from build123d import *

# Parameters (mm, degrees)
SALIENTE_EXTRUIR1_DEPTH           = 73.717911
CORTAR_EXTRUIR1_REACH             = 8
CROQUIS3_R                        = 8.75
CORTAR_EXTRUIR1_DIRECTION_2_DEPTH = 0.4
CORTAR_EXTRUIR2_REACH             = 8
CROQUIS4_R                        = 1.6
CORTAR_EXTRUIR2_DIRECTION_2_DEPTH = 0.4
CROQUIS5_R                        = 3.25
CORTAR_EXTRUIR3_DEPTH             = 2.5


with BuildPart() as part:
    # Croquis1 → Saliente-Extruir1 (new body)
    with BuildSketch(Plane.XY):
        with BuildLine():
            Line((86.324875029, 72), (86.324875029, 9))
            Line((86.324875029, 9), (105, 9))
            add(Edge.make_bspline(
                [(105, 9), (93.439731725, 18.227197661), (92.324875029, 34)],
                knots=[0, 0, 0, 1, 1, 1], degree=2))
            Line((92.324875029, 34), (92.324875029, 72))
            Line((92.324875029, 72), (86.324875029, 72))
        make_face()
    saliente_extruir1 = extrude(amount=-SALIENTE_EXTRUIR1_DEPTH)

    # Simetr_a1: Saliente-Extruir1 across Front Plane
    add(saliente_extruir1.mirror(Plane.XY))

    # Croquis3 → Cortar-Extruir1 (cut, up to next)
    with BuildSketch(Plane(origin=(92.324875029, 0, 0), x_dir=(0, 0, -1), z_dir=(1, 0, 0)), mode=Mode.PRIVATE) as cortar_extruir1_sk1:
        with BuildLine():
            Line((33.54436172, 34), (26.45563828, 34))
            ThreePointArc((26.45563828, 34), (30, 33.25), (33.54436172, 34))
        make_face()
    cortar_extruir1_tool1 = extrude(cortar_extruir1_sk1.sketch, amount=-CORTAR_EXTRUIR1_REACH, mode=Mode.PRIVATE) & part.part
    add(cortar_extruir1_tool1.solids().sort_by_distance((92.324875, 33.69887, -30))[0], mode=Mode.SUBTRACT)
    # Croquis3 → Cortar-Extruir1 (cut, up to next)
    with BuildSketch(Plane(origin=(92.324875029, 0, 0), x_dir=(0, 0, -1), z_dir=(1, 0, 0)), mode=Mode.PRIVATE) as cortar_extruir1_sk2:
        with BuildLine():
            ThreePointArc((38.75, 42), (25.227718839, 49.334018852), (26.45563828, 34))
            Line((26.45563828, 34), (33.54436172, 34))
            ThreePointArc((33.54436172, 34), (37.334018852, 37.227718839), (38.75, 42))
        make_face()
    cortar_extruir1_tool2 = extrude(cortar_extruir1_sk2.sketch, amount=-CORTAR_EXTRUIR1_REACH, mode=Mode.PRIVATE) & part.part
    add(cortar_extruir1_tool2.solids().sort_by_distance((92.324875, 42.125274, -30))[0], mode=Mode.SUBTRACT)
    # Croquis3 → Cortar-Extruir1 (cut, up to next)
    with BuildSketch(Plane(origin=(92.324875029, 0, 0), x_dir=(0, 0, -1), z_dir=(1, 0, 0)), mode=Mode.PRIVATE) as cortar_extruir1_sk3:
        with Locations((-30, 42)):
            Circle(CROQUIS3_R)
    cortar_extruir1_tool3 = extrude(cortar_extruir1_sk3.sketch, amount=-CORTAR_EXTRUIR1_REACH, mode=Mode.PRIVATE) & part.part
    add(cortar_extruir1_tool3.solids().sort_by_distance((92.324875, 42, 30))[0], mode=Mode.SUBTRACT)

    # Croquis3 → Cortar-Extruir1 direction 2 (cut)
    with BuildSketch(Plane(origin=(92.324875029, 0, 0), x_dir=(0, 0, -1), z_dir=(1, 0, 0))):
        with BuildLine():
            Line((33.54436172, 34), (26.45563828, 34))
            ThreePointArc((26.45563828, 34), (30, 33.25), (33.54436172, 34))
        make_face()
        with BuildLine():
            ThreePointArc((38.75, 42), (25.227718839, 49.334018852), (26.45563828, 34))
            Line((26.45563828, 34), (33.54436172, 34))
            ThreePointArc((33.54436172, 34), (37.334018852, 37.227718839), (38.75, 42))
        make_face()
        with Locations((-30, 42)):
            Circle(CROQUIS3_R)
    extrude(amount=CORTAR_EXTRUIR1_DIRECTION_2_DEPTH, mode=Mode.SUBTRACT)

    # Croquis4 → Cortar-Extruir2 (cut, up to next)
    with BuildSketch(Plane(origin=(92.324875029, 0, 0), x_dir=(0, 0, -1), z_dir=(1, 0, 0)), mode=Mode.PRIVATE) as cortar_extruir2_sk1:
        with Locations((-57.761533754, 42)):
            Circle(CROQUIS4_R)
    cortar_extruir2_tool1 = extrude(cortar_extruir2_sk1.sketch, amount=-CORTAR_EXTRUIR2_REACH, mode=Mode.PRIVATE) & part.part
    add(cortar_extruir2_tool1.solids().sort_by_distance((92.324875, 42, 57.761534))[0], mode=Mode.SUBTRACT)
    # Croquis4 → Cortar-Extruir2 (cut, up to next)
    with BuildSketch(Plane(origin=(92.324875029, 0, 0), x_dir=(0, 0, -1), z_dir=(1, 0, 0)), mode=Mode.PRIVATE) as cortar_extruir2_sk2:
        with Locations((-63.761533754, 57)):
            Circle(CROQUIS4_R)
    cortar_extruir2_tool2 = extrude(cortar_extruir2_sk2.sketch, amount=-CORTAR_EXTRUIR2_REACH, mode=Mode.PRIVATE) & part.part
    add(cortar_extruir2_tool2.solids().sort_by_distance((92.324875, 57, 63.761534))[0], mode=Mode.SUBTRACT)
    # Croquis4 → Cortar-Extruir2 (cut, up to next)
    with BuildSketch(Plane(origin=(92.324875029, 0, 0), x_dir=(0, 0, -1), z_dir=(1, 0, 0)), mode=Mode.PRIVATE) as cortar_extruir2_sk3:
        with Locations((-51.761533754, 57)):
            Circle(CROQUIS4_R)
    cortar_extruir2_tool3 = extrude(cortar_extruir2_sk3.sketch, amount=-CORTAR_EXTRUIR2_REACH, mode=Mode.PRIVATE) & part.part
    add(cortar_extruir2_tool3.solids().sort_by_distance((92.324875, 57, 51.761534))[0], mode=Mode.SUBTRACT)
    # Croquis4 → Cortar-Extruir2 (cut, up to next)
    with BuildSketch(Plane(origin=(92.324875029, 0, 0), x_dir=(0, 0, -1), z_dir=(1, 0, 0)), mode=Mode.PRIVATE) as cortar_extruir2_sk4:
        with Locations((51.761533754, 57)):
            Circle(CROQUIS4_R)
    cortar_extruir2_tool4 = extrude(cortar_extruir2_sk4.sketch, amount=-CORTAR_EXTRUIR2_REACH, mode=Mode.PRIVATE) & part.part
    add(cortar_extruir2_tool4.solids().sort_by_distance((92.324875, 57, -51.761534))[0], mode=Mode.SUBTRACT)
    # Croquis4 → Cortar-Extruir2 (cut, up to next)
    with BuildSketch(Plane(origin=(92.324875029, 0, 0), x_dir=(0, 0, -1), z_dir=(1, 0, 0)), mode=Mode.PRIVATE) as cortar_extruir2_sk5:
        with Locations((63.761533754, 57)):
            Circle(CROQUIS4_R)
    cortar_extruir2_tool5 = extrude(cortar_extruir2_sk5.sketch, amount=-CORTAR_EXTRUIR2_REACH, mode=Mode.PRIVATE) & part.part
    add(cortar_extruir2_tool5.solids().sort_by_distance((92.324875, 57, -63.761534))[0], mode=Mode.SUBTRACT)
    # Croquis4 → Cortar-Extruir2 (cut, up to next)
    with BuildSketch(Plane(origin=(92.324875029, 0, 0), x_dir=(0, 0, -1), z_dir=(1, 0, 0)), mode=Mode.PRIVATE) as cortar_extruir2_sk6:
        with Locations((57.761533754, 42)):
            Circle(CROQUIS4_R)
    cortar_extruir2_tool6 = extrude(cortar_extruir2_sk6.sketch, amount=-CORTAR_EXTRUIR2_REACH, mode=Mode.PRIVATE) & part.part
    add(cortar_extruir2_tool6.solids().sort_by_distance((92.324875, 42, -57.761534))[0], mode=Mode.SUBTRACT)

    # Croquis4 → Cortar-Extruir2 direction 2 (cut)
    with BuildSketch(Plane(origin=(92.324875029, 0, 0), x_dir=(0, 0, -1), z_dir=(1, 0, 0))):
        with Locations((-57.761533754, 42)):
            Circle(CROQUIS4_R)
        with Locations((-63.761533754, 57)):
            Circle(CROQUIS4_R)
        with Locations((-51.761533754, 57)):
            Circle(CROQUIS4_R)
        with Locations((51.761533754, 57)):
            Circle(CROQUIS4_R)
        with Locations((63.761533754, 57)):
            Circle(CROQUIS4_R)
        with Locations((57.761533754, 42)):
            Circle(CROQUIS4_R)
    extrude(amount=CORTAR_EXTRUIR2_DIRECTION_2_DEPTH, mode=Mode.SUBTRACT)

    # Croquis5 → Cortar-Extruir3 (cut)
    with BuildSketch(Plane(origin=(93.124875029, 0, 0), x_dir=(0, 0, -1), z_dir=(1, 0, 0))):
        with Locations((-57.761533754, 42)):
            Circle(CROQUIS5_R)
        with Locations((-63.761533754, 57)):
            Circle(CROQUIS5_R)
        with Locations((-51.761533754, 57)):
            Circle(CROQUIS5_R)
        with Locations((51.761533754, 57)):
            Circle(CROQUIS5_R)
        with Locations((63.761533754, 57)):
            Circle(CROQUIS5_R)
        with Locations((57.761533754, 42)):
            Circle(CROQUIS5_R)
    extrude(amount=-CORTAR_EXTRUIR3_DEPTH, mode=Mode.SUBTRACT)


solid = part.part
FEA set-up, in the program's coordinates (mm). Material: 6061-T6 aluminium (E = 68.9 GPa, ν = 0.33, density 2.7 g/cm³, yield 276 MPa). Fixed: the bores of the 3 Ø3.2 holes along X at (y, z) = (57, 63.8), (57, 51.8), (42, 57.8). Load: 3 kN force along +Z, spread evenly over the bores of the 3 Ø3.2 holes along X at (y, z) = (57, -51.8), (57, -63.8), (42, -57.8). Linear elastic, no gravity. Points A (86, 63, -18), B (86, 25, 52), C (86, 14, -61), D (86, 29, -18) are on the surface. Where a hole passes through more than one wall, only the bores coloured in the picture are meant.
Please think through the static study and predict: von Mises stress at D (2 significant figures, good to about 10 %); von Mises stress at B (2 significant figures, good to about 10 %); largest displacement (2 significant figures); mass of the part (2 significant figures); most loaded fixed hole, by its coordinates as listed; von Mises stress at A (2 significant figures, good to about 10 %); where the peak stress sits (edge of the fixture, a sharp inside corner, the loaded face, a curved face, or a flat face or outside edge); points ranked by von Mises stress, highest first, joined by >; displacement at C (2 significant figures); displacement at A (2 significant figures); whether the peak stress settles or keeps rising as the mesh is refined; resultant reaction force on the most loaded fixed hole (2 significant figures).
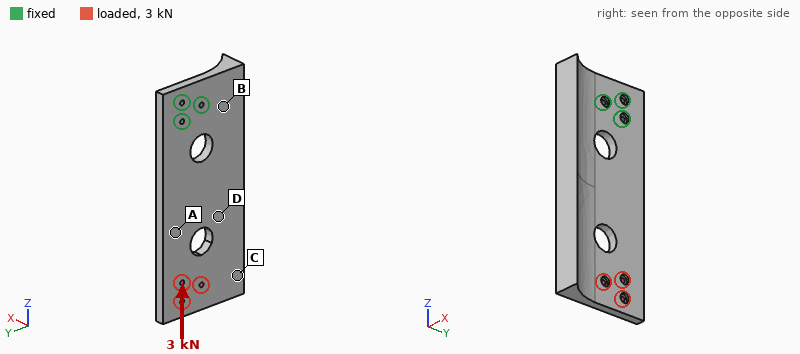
11 MPa
7.0 MPa
0.15 mm
180 g
(57, 51.8)
20 MPa
edge of the fixture
A > D > B > C
0.11 mm
0.048 mm
keeps rising
1.4 kN
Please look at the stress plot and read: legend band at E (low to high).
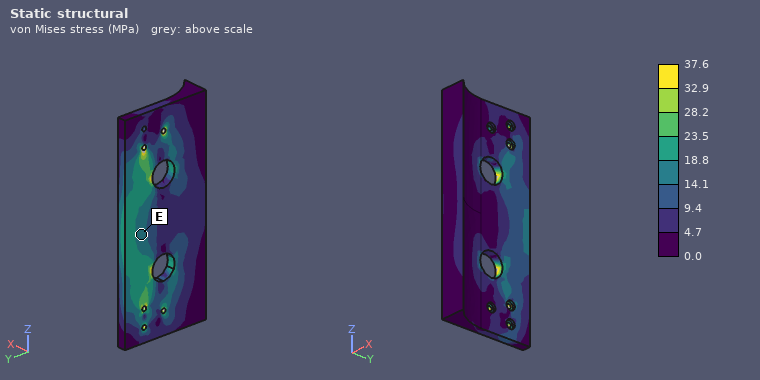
14.1 to 18.8 MPa
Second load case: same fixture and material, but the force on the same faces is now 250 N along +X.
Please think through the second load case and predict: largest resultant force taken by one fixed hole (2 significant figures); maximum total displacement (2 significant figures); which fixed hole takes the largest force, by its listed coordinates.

1.3 kN
1.3 mm
(57, 51.8)
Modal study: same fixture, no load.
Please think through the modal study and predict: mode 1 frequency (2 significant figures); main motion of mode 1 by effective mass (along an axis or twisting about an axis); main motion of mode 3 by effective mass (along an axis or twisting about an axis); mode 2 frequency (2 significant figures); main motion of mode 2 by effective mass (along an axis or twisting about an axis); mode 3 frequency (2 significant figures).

300 Hz
along X
along Y
1000 Hz
twisting about Z
1300 Hz
